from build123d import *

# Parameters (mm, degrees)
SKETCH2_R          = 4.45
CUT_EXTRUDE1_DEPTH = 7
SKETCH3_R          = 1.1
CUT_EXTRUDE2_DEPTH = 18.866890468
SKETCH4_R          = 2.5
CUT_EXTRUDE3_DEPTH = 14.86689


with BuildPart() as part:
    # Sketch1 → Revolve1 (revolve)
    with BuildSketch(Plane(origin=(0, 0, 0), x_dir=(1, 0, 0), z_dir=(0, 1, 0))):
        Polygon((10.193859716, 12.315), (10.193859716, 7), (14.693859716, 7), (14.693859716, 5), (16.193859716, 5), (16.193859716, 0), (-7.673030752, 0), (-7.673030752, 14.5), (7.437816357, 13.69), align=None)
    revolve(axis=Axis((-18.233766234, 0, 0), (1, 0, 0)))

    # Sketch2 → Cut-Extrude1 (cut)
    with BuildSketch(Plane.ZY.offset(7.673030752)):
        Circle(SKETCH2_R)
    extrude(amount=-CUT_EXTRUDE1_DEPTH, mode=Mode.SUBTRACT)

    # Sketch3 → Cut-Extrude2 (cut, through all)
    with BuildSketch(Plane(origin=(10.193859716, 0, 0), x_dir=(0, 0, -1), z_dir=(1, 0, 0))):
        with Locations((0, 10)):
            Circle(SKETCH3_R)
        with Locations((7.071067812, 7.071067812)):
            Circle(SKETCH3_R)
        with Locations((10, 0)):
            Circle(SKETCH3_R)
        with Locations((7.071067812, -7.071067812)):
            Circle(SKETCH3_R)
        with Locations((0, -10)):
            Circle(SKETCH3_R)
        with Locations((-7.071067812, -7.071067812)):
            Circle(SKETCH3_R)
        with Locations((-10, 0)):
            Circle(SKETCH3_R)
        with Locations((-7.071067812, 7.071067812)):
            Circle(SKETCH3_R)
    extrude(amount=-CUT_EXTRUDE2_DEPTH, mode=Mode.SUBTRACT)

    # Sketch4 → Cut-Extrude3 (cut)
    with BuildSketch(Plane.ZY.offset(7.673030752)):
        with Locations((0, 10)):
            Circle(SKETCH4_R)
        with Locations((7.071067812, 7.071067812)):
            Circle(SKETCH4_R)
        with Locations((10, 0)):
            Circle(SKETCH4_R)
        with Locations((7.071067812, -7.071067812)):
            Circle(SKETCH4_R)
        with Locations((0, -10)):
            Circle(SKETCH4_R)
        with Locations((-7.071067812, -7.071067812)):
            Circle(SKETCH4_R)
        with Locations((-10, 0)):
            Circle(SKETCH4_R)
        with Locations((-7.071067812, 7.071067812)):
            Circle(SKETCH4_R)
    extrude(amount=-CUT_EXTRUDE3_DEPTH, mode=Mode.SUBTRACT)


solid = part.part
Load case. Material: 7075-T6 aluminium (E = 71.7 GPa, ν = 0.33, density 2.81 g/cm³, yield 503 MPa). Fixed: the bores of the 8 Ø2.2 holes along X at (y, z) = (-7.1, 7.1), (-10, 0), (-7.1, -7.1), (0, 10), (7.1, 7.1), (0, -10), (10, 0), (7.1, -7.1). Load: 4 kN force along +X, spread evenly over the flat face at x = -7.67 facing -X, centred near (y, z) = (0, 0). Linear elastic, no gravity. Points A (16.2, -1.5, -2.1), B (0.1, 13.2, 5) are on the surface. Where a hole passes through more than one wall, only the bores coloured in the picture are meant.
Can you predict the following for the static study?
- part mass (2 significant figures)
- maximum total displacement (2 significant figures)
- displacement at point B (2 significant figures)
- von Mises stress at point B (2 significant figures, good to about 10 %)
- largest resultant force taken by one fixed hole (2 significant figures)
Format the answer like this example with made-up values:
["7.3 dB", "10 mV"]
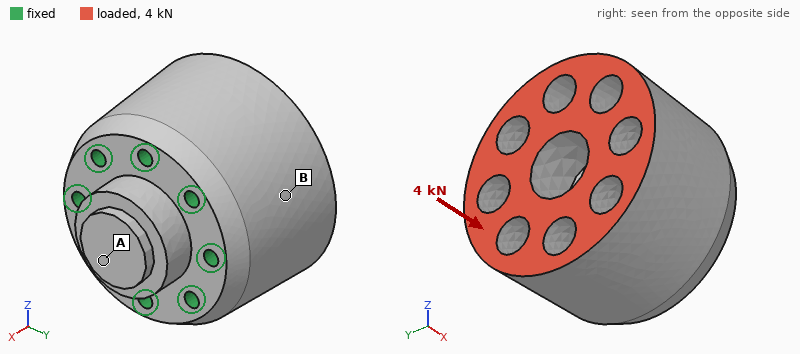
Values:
["25 g", "4.0 µm", "2.8 µm", "10 MPa", "500 N"]
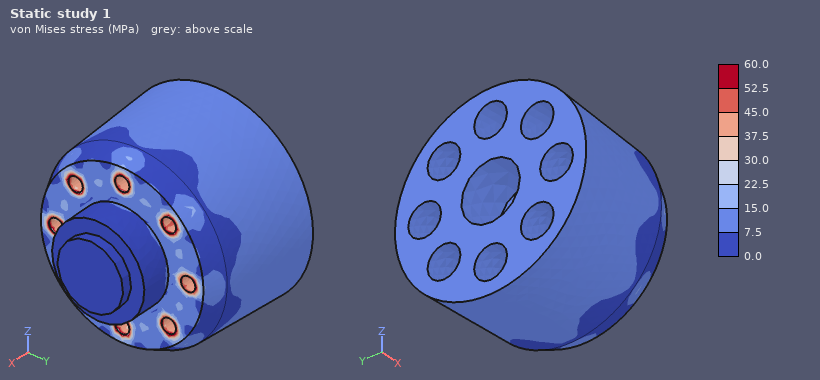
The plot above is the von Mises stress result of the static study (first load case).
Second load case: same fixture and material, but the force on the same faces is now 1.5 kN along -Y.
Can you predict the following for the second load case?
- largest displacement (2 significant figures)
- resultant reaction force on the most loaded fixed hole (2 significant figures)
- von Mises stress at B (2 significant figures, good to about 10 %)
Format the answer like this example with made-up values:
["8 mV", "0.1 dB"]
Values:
["9.9 µm", "600 N", "8.7 MPa"]
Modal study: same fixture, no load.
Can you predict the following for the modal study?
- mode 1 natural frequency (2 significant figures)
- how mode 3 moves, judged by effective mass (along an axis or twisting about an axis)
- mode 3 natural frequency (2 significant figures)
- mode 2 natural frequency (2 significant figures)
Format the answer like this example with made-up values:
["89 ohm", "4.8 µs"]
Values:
["25 kHz", "twisting about X", "38 kHz", "25 kHz"]
